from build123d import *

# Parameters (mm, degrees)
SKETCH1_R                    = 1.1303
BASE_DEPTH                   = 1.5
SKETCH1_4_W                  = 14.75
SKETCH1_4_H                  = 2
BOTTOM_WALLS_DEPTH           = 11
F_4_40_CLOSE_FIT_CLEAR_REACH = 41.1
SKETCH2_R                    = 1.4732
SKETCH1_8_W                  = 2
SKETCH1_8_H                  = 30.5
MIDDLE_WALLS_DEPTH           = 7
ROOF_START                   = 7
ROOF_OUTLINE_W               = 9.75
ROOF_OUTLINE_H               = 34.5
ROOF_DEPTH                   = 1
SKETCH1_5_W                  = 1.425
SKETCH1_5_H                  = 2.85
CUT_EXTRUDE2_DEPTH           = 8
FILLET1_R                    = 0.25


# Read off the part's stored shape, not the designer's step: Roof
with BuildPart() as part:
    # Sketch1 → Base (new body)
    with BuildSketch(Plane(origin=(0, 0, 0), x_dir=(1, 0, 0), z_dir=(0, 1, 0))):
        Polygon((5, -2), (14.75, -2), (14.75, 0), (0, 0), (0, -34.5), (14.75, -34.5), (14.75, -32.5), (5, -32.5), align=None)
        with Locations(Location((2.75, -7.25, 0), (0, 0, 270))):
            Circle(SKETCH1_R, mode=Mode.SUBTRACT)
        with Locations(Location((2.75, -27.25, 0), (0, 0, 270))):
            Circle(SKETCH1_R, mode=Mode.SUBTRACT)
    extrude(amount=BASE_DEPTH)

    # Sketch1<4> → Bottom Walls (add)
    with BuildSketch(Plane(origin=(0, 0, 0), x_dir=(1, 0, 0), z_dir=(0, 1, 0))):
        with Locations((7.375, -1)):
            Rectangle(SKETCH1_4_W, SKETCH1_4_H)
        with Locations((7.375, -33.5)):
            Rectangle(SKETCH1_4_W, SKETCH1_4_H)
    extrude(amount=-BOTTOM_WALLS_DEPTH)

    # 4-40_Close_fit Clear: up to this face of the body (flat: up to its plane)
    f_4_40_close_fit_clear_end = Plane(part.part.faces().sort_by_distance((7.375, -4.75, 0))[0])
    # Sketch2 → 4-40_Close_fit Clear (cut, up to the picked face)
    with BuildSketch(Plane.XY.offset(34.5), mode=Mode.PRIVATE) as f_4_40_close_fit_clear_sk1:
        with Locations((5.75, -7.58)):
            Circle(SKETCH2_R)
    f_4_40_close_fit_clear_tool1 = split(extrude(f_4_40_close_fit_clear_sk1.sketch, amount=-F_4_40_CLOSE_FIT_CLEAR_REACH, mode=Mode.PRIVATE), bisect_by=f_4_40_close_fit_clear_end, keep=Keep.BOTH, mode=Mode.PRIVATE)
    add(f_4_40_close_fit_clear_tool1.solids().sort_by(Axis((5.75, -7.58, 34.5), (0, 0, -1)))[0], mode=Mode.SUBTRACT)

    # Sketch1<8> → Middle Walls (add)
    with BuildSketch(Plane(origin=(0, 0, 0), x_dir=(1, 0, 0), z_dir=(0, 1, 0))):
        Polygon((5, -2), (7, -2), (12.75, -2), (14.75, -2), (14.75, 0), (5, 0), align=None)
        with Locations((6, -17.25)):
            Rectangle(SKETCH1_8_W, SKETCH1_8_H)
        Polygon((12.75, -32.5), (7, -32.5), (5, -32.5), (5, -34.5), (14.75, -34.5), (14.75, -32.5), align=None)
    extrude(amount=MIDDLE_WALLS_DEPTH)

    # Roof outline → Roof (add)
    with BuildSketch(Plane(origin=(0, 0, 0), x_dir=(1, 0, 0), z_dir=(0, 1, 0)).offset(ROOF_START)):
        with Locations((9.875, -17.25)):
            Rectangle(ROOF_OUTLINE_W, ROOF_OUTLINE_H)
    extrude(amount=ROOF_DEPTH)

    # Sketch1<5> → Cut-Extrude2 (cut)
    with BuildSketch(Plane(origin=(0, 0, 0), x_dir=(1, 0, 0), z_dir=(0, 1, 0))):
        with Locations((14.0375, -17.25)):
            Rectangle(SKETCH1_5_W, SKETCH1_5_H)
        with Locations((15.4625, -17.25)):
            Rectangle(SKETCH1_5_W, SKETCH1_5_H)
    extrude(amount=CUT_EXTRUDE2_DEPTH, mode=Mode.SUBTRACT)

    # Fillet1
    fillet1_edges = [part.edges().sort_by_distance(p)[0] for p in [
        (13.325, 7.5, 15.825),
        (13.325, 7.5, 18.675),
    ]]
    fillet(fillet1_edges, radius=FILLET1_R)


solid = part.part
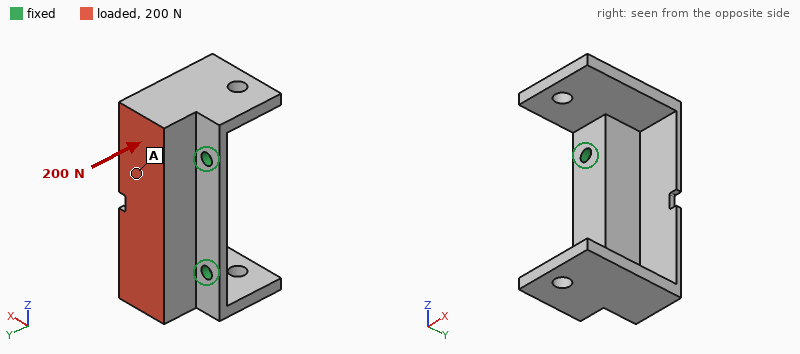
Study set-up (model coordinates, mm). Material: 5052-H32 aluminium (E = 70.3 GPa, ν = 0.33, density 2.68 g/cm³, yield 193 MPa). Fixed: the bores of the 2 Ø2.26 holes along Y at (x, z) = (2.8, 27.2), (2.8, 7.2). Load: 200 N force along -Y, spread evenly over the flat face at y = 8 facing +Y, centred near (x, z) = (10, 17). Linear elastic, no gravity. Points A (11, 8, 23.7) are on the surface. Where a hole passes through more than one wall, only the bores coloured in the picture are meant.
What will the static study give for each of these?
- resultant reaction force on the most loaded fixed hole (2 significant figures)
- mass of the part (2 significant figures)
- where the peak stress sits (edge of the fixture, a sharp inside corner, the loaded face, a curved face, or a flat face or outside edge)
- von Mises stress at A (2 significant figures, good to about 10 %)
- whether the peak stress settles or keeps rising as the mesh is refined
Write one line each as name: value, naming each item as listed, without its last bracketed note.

resultant reaction force on the most loaded fixed hole: 100 N
mass of the part: 5.1 g
where the peak stress sits: edge of the fixture
von Mises stress at A: 23 MPa
whether the peak stress settles or keeps rising as the mesh is refined: keeps rising
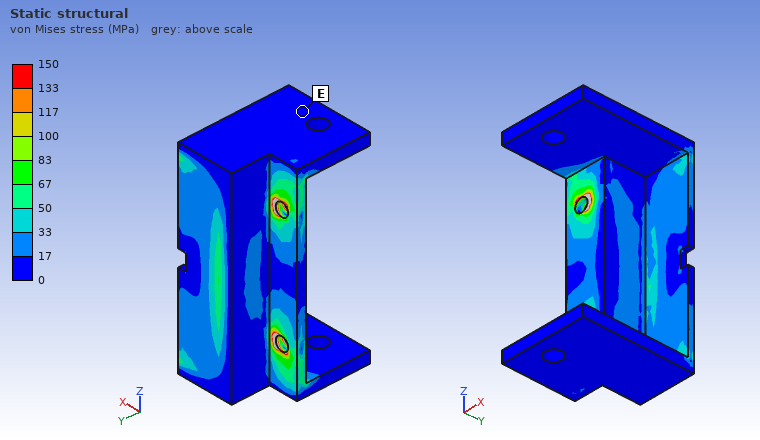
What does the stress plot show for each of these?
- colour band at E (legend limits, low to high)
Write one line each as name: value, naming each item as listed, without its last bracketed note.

colour band at E: 0 to 17 MPa
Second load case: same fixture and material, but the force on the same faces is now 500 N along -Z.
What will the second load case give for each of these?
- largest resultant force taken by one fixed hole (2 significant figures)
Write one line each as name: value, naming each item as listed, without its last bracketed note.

largest resultant force taken by one fixed hole: 330 N
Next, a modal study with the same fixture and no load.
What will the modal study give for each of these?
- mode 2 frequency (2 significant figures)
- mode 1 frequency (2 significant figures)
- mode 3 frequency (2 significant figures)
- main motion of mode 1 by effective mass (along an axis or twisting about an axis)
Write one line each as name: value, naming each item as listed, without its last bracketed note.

mode 2 frequency: 4900 Hz
mode 1 frequency: 4300 Hz
mode 3 frequency: 7100 Hz
main motion of mode 1 by effective mass: along Y
